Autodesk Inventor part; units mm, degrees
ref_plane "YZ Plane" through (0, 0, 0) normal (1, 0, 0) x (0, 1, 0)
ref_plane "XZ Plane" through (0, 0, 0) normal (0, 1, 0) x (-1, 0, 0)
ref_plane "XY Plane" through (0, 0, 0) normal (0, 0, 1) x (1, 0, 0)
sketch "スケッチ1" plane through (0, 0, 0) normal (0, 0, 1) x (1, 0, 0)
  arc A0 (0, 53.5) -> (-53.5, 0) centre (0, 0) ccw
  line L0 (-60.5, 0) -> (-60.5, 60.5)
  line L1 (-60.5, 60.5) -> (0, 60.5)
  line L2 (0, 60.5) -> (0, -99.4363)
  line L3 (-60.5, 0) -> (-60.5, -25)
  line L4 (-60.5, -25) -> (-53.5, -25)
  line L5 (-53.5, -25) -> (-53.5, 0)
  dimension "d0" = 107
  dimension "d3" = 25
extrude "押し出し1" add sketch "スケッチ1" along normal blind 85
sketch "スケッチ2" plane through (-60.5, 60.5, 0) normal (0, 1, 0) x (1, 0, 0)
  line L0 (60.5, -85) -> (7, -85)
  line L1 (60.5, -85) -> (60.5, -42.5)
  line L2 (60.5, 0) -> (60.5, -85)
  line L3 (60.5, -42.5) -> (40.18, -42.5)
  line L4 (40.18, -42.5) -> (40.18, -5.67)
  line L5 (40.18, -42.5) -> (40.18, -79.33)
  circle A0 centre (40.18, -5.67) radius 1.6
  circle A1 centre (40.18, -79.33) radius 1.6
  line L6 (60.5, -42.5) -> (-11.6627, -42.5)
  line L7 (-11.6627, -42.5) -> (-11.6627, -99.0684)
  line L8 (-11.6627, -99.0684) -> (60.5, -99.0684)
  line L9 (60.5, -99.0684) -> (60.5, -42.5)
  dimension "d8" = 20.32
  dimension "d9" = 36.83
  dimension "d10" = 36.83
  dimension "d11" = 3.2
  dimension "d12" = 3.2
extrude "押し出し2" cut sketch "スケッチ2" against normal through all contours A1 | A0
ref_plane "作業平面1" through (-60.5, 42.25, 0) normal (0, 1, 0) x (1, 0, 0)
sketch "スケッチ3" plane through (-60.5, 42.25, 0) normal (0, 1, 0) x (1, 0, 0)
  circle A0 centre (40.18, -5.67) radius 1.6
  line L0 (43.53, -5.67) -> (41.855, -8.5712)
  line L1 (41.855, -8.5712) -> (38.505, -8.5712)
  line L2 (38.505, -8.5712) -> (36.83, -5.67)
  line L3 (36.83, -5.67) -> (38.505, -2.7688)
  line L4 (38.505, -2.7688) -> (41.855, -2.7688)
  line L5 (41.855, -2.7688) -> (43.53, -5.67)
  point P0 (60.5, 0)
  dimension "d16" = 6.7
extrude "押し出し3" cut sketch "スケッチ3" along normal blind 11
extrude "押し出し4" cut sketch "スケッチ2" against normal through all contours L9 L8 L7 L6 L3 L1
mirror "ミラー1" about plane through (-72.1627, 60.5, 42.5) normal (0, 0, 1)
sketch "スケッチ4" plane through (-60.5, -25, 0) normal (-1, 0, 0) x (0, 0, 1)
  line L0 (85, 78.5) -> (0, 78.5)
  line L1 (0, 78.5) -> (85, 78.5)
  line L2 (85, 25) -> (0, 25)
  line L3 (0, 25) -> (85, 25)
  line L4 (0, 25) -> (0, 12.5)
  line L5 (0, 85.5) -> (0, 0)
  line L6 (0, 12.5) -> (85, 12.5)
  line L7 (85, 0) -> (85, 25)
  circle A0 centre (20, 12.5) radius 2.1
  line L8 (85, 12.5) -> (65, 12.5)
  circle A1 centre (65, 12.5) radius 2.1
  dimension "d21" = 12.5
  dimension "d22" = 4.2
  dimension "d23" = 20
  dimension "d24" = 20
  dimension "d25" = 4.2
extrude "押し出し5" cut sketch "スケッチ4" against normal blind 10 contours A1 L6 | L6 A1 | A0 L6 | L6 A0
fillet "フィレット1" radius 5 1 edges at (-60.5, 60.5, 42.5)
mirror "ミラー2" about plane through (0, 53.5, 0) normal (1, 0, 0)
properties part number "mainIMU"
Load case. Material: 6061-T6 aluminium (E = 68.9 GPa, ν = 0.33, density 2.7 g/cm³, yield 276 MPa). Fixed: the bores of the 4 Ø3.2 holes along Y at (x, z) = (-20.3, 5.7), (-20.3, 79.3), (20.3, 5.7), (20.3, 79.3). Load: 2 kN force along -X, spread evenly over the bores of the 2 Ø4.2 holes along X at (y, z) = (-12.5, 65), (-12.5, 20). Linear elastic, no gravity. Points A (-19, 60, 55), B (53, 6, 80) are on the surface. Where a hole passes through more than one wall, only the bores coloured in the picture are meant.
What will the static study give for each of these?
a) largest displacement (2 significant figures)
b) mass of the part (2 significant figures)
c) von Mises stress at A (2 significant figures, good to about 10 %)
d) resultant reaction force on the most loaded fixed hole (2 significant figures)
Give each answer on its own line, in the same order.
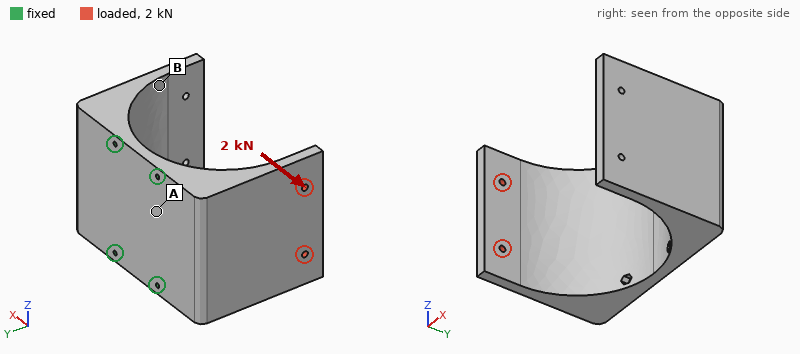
0.68 mm
720 g
50 MPa
1.3 kN
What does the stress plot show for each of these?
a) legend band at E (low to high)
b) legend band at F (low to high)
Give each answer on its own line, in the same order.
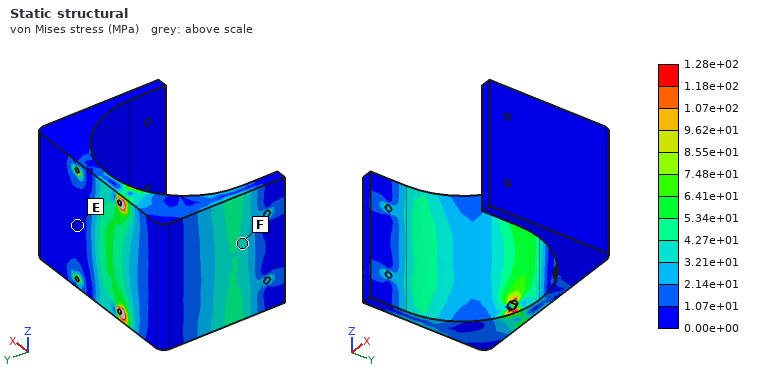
0.00e+00 to 1.07e+01 MPa
3.21e+01 to 4.27e+01 MPa
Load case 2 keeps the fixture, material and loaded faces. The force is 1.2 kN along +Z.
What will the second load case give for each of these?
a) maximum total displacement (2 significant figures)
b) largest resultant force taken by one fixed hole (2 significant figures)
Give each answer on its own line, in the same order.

40 µm
1.4 kN
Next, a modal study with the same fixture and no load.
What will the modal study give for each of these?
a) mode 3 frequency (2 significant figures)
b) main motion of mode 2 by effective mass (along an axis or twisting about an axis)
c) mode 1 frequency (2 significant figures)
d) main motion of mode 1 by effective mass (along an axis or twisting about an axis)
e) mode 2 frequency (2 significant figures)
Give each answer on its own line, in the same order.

3200 Hz
along X
950 Hz
along Y
1100 Hz
